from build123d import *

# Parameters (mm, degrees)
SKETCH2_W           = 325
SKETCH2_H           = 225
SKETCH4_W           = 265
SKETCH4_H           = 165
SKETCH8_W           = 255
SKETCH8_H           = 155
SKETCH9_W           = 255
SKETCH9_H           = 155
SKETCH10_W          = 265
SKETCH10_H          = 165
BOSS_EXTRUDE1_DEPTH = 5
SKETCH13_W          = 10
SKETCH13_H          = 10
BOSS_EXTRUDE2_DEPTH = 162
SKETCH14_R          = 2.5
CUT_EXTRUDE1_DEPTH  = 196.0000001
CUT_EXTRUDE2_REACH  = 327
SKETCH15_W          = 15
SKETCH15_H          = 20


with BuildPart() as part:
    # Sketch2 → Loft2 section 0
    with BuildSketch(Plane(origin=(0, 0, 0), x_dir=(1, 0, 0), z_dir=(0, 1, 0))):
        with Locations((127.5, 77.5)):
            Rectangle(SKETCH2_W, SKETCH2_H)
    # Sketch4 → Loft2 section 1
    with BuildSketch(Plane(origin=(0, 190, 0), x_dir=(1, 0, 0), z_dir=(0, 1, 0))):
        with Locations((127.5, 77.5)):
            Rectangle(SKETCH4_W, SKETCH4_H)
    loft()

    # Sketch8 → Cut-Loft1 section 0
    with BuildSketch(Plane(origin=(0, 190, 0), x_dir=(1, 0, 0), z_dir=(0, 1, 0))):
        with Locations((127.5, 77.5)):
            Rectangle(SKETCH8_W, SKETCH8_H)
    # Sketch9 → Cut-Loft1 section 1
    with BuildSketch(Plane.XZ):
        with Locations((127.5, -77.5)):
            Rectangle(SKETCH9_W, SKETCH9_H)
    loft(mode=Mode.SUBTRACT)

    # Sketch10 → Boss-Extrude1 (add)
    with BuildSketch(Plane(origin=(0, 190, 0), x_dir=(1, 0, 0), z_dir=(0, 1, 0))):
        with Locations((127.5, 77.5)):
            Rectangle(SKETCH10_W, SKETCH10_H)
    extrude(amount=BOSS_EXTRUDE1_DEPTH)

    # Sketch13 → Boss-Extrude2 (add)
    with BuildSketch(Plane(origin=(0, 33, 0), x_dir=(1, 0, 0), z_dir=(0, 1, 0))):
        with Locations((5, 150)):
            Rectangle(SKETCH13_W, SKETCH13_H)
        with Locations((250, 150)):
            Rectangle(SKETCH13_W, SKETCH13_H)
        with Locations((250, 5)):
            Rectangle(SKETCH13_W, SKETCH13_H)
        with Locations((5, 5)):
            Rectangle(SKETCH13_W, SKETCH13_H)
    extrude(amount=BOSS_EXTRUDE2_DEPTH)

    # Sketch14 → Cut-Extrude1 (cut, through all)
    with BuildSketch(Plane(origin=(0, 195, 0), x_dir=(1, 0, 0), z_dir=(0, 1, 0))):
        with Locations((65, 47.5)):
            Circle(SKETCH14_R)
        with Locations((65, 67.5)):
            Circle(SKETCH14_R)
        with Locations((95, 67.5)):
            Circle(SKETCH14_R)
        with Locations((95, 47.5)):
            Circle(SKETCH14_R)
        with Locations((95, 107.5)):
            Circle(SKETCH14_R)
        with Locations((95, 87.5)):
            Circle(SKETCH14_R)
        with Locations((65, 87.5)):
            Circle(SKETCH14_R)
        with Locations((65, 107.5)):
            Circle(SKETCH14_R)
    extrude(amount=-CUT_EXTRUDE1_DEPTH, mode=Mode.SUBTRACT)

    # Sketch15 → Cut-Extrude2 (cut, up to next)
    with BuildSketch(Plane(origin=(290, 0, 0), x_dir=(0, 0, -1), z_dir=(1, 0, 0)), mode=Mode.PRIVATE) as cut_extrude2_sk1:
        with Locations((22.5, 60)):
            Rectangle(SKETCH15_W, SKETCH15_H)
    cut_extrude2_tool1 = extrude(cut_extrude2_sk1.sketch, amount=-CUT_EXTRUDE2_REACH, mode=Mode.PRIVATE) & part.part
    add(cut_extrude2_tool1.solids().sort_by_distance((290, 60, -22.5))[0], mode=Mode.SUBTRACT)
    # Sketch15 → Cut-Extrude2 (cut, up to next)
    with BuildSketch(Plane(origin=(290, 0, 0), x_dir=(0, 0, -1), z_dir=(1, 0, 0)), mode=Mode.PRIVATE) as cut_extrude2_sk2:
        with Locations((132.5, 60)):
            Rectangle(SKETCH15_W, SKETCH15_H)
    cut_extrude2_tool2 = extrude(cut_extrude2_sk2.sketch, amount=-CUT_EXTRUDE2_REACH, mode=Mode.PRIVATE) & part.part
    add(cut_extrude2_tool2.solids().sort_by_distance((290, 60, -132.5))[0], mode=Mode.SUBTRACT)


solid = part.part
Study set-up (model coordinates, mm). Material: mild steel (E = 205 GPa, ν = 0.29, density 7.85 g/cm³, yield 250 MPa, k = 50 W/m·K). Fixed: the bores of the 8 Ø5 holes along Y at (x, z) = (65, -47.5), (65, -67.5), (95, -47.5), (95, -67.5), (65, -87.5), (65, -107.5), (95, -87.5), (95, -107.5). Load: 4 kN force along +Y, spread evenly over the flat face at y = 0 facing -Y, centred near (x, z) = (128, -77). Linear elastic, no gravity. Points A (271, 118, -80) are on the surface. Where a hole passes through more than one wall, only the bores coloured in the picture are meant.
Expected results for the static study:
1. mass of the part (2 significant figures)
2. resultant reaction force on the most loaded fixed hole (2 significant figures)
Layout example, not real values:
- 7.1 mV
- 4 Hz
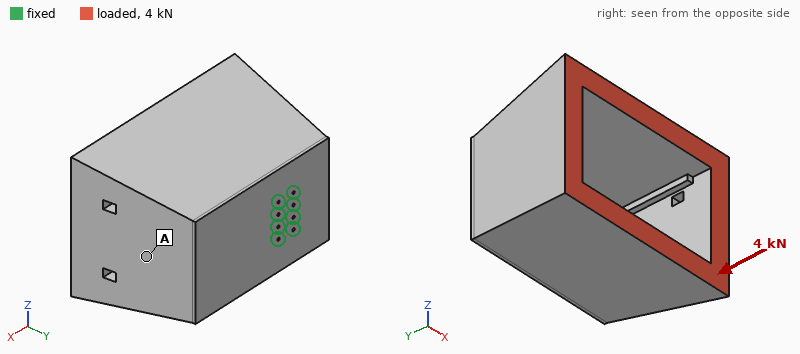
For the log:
- 29 kg
- 3.1 kN
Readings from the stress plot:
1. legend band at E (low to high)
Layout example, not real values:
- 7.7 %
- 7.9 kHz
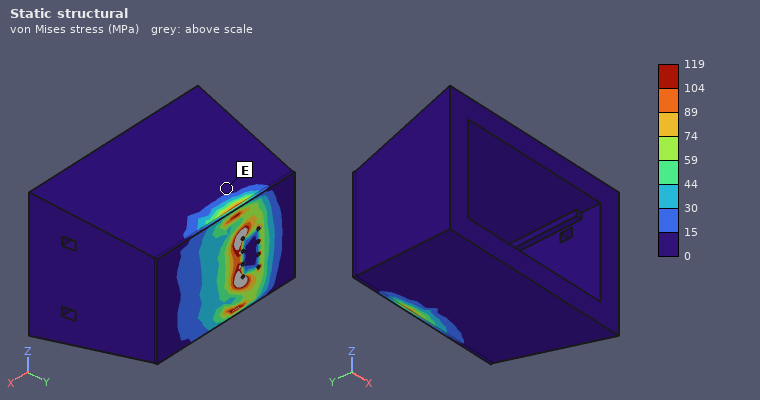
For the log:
- 0 to 15 MPa
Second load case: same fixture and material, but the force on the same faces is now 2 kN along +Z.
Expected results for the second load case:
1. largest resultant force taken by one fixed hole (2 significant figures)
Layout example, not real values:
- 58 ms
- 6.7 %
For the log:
- 2.7 kN
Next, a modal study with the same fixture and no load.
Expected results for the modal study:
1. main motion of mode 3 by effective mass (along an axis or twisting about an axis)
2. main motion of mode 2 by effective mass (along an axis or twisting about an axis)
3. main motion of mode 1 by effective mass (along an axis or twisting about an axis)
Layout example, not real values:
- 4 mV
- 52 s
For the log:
- along Y
- along Z
- along X
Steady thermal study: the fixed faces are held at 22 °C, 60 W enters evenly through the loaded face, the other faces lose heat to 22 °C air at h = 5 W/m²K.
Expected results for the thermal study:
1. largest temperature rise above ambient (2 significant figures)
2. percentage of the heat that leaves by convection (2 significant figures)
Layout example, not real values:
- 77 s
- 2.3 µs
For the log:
- 26 K
- 71 %
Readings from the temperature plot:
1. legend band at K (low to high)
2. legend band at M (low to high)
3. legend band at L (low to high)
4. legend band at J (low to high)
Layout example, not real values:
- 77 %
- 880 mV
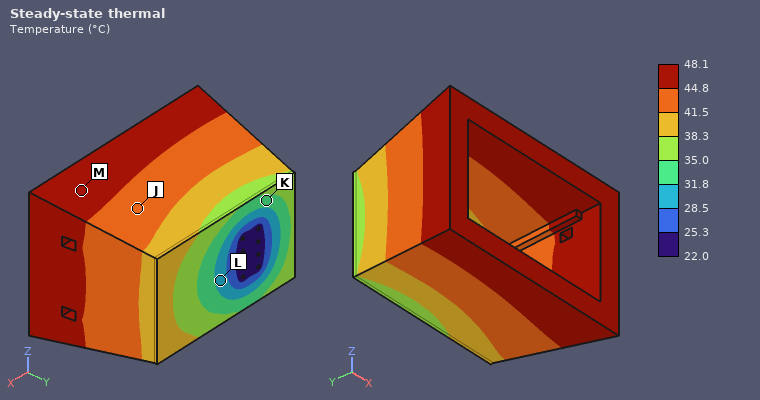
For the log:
- 31.8 to 35.0 °C
- 44.8 to 48.1 °C
- 28.5 to 31.8 °C
- 41.5 to 44.8 °C
